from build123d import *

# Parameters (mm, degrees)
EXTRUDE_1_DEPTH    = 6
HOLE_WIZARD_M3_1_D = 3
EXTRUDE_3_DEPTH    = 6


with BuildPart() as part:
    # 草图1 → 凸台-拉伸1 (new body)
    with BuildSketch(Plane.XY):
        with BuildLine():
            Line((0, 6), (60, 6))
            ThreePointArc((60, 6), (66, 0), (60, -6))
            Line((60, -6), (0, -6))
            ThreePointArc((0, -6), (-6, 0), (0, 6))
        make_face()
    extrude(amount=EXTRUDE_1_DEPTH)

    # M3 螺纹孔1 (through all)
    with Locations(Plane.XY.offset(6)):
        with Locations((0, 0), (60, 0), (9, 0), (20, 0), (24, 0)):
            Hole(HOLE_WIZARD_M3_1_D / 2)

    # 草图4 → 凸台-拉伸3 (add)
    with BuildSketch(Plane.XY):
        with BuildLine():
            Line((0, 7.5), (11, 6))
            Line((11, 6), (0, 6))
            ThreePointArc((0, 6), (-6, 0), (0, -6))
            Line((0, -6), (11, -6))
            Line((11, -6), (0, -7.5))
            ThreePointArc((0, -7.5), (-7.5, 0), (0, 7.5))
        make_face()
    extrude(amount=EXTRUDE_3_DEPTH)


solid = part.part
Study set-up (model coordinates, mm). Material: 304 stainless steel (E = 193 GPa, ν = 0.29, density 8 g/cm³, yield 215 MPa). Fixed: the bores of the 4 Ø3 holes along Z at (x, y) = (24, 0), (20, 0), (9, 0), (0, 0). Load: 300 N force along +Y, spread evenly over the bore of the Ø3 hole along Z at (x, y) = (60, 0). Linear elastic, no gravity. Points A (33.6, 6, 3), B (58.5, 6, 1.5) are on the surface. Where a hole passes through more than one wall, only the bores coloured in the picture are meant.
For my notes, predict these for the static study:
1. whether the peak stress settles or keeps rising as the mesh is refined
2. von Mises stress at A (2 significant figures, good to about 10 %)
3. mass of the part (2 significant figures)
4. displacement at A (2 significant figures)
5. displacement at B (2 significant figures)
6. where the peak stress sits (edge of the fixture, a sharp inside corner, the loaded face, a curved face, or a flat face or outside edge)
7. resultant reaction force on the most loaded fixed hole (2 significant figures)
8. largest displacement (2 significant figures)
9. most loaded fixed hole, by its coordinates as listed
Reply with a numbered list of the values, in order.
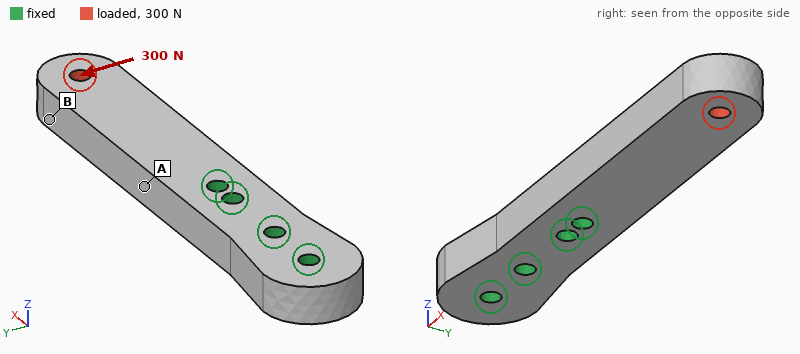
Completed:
1. keeps rising
2. 55 MPa
3. 41 g
4. 7.6 µm
5. 38 µm
6. edge of the fixture
7. 1.1 kN
8. 48 µm
9. (24, 0)
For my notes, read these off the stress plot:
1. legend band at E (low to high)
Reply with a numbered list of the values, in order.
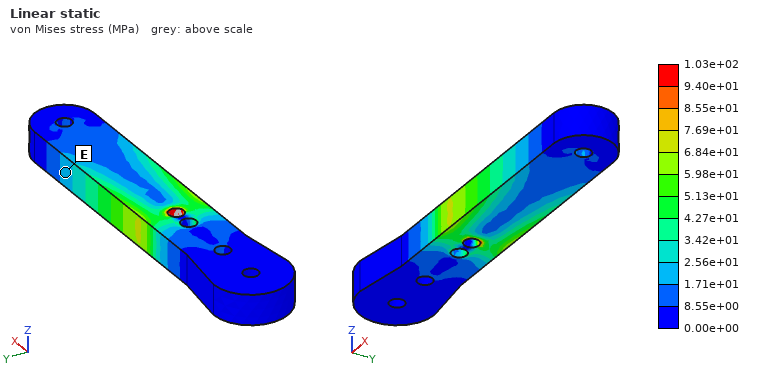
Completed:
1. 1.71e+01 to 2.56e+01 MPa
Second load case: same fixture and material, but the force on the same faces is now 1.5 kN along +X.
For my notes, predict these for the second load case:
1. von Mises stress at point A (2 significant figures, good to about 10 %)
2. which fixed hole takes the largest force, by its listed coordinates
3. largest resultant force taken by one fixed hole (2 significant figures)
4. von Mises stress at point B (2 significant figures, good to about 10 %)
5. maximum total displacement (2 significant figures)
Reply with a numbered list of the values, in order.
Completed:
1. 20 MPa
2. (24, 0)
3. 1.1 kN
4. 8.3 MPa
5. 4.7 µm
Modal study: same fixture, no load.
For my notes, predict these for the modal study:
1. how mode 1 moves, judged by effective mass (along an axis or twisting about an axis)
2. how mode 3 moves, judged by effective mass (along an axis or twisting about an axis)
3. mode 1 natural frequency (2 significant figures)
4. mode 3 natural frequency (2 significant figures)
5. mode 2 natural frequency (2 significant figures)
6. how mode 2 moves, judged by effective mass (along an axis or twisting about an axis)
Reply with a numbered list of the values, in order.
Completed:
1. along Z
2. twisting about X
3. 2900 Hz
4. 14 kHz
5. 4700 Hz
6. along Y
